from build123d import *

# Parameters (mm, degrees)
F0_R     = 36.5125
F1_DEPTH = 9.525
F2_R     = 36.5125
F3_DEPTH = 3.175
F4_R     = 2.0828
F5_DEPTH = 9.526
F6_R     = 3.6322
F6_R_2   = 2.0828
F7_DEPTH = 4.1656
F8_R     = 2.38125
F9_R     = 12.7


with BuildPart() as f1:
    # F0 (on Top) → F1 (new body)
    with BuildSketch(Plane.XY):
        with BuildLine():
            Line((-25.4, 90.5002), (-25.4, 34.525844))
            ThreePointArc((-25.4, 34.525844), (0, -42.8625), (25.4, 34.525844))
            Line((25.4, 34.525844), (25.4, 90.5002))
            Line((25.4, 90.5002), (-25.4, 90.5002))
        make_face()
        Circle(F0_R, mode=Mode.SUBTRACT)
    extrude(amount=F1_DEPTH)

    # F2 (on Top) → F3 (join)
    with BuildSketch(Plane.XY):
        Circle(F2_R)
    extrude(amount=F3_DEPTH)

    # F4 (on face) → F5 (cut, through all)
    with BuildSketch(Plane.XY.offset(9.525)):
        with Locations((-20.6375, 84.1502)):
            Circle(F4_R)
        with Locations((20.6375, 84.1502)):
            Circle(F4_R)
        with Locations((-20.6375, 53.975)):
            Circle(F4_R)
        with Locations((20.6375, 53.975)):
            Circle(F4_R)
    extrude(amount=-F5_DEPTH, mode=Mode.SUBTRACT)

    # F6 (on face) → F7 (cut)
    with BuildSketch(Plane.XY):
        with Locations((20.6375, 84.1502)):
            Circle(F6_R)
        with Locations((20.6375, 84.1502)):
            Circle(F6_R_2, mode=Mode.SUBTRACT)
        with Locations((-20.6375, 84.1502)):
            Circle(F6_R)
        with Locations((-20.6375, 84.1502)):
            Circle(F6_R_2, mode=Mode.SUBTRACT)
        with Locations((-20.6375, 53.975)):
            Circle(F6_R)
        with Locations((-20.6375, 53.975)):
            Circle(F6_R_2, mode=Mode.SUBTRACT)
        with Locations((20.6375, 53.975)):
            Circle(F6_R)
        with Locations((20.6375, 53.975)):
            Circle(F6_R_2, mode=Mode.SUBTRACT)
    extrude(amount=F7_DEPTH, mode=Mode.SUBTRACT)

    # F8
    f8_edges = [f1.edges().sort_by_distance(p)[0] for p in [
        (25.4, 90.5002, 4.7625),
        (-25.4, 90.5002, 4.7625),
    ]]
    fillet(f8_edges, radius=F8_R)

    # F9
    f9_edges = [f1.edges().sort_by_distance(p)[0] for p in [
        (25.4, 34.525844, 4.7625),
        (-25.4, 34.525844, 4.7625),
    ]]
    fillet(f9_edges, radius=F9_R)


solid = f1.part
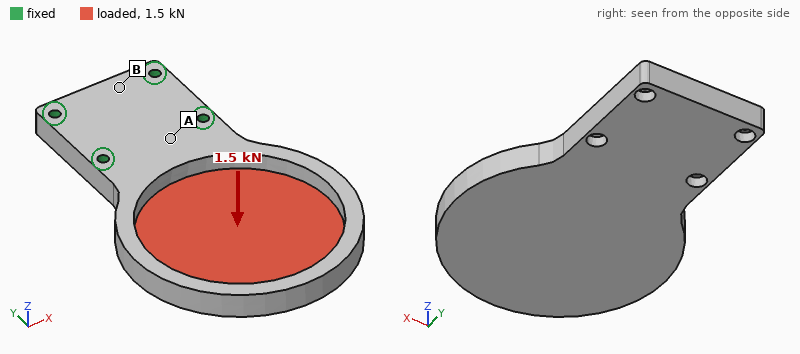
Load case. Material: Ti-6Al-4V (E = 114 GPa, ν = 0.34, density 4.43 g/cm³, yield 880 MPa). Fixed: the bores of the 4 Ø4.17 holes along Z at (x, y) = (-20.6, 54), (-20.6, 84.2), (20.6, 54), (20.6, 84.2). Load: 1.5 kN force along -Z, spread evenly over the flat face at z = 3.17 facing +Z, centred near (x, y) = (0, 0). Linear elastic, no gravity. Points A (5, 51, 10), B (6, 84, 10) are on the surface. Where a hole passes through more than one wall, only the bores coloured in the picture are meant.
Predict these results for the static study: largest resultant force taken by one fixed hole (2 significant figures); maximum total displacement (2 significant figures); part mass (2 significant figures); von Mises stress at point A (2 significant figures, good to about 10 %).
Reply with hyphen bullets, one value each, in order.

- 2.2 kN
- 1.1 mm
- 230 g
- 61 MPa
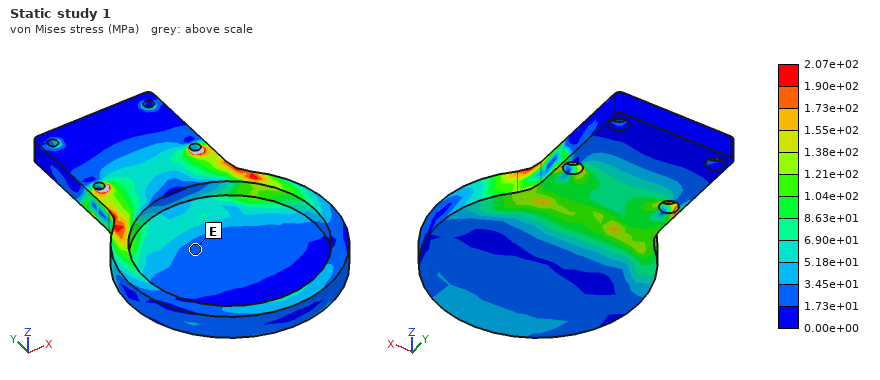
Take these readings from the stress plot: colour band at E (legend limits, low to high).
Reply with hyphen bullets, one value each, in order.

- 1.73e+01 to 3.45e+01 MPa
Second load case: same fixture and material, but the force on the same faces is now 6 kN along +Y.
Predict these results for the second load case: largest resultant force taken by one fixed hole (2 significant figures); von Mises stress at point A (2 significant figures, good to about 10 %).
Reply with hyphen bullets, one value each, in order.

- 2.2 kN
- 9.9 MPa
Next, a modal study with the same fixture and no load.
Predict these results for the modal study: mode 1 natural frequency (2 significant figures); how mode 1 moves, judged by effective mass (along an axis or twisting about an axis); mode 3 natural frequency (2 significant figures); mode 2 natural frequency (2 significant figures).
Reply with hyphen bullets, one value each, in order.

- 640 Hz
- along Z
- 3200 Hz
- 1500 Hz
